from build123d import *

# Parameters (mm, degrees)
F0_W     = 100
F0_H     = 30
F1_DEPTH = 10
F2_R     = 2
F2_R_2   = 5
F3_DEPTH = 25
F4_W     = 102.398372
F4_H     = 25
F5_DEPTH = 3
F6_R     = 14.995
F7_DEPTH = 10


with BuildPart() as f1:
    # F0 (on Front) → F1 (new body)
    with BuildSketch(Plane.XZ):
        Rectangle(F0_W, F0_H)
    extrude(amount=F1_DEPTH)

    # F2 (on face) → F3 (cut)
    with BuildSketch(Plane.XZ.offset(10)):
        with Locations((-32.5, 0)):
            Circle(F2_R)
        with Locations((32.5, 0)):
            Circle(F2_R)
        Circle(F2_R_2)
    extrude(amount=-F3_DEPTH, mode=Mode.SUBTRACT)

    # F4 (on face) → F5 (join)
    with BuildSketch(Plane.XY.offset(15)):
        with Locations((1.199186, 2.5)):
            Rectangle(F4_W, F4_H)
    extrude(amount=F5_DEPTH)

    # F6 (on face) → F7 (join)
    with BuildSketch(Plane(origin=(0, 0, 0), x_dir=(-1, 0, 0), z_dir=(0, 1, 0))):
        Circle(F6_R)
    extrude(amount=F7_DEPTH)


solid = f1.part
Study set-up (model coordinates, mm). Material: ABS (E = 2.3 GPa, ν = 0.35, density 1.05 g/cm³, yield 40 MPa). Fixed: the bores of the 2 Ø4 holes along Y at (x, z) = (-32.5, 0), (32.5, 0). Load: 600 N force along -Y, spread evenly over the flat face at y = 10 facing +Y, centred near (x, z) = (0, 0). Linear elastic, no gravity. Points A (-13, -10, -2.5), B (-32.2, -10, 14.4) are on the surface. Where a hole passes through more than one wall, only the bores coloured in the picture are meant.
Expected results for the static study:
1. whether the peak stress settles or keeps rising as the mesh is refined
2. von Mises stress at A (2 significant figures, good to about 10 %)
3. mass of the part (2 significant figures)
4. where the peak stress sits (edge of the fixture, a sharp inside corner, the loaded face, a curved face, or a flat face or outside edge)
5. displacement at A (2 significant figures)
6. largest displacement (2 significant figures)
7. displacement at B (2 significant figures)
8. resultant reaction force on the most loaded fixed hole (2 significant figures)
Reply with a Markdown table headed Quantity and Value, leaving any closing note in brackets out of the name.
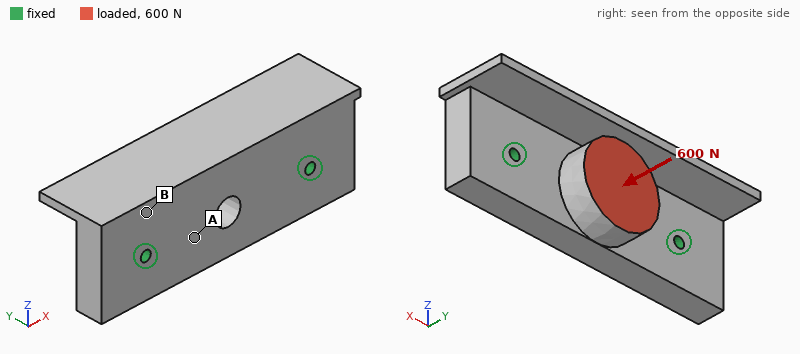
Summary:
| Quantity | Value |
|---|---|
| whether the peak stress settles or keeps rising as the mesh is refined | keeps rising |
| von Mises stress at A | 2.8 MPa |
| mass of the part | 46 g |
| where the peak stress sits | edge of the fixture |
| displacement at A | 0.098 mm |
| largest displacement | 0.14 mm |
| displacement at B | 0.028 mm |
| resultant reaction force on the most loaded fixed hole | 330 N |
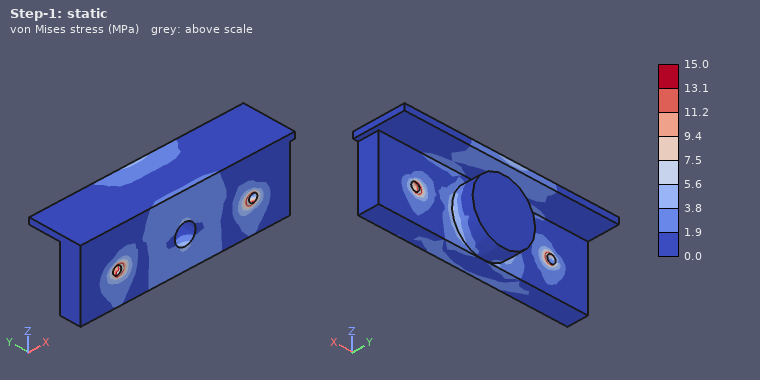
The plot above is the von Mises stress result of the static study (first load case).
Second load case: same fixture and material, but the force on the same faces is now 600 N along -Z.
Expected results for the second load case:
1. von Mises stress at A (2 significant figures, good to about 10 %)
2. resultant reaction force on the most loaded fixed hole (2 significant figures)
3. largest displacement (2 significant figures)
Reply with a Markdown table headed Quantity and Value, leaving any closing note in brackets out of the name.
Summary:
| Quantity | Value |
|---|---|
| von Mises stress at A | 2.8 MPa |
| resultant reaction force on the most loaded fixed hole | 310 N |
| largest displacement | 0.37 mm |
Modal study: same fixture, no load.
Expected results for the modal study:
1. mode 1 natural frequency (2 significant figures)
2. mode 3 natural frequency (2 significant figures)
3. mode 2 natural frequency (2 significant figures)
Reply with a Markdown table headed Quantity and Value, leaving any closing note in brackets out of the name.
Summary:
| Quantity | Value |
|---|---|
| mode 1 natural frequency | 1900 Hz |
| mode 3 natural frequency | 2600 Hz |
| mode 2 natural frequency | 2500 Hz |
